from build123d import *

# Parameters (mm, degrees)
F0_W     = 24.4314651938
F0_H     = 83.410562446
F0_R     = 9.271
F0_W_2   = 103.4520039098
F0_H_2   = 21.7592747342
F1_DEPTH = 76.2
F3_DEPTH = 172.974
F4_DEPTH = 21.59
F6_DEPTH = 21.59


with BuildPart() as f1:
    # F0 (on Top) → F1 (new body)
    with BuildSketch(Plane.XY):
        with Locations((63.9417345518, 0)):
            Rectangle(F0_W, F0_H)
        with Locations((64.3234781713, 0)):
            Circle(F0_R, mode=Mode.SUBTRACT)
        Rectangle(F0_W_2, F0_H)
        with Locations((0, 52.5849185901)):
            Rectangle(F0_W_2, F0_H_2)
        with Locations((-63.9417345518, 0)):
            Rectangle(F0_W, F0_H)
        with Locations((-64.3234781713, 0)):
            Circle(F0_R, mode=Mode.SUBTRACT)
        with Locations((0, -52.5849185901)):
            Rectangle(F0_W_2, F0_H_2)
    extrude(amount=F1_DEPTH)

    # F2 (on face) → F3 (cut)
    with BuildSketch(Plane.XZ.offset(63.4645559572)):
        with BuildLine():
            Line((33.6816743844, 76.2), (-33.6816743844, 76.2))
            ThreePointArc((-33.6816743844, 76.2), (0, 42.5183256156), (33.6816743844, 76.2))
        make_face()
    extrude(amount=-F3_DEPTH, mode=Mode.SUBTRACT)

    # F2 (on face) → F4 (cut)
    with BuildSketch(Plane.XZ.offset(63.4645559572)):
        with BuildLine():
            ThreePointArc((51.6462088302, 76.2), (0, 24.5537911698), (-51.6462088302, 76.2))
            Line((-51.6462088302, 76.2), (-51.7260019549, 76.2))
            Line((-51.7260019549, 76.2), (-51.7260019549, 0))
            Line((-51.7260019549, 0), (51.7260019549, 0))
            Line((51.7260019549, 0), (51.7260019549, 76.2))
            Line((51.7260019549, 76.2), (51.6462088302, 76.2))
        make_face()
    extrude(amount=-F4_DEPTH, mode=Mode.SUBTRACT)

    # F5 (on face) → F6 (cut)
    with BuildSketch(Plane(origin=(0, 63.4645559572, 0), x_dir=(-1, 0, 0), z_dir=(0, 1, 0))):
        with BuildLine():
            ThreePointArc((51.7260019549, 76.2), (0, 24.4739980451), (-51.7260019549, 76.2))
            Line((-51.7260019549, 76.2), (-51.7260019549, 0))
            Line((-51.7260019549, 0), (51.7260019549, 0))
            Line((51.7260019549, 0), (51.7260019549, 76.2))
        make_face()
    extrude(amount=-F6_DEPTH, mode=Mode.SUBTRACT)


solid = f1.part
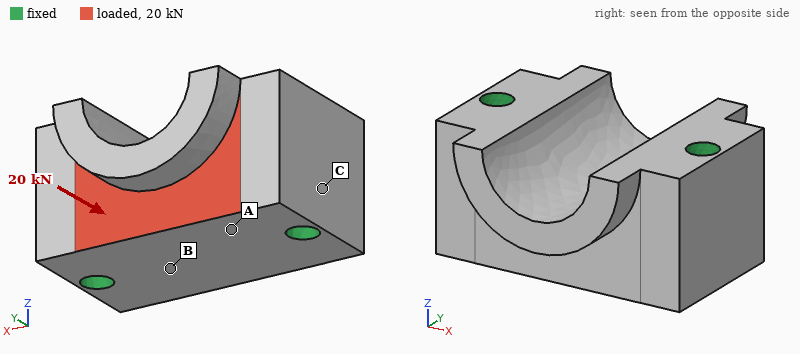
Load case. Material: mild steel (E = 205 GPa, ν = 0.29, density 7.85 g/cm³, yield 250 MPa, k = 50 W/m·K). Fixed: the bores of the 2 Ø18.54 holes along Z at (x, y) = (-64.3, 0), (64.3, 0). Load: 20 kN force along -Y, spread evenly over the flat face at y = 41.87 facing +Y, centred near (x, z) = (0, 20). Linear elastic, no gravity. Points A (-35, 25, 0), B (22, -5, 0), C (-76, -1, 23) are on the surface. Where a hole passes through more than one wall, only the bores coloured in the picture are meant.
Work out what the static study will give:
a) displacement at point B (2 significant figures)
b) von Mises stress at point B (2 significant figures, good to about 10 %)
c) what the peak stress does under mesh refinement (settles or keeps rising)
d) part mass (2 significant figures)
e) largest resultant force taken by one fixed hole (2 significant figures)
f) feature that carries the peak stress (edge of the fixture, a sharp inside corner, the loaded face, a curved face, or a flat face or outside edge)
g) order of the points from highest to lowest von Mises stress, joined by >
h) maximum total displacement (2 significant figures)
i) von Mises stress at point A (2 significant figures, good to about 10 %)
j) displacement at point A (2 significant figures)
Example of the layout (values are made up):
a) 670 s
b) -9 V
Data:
a) 1.7 µm
b) 3.5 MPa
c) keeps rising
d) 6.9 kg
e) 10 kN
f) edge of the fixture
g) A > B > C
h) 3.2 µm
i) 6.4 MPa
j) 1.9 µm
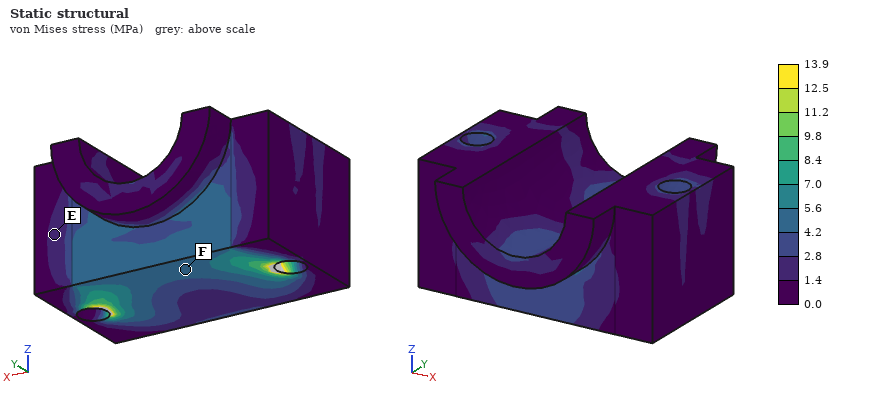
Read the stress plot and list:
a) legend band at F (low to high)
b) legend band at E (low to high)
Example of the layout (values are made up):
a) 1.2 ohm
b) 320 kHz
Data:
a) 4.2 to 5.6 MPa
b) 1.4 to 2.8 MPa
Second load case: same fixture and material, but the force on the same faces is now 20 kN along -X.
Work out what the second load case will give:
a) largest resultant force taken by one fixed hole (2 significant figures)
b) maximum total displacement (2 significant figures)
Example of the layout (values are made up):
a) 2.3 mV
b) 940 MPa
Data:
a) 12 kN
b) 2.1 µm
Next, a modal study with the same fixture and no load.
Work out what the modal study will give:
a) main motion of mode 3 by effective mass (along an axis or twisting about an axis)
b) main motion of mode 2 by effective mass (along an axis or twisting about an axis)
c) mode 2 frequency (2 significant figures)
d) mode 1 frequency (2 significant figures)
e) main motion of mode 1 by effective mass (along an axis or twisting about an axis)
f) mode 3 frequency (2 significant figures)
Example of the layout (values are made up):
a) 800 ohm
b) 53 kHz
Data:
a) along Y
b) along Z
c) 8900 Hz
d) 8300 Hz
e) along Y
f) 9700 Hz
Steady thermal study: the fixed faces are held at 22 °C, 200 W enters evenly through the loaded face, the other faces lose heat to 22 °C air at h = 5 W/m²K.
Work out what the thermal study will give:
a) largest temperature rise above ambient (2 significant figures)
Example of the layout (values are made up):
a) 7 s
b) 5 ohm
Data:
a) 40 K
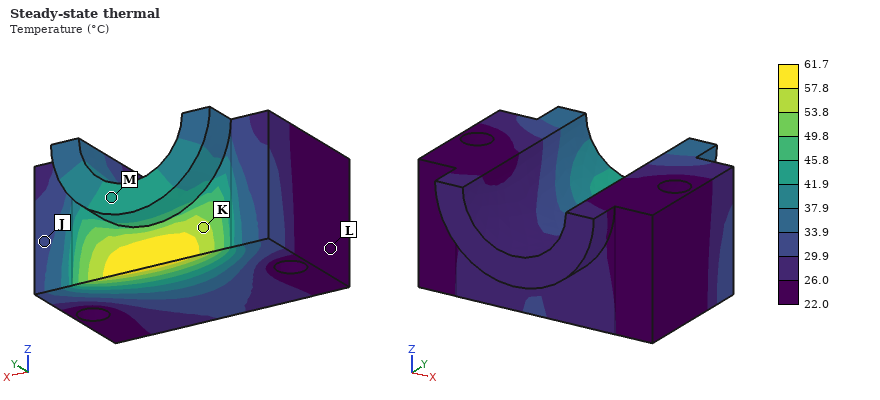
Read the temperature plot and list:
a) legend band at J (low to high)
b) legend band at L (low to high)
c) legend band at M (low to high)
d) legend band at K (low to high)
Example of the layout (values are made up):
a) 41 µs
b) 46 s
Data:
a) 29.9 to 33.9 °C
b) 22.0 to 26.0 °C
c) 41.9 to 45.8 °C
d) 53.8 to 57.8 °C
